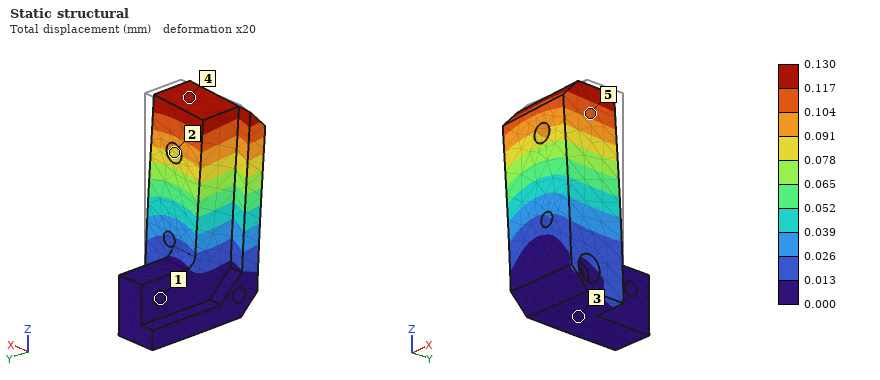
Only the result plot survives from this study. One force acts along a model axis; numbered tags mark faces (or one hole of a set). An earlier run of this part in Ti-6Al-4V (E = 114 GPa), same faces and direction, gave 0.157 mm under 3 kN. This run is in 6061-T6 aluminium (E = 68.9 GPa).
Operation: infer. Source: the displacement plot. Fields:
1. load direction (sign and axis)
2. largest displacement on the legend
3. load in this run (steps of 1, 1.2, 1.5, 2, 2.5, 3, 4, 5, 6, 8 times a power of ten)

-X
0.130 mm
1.5 kN
